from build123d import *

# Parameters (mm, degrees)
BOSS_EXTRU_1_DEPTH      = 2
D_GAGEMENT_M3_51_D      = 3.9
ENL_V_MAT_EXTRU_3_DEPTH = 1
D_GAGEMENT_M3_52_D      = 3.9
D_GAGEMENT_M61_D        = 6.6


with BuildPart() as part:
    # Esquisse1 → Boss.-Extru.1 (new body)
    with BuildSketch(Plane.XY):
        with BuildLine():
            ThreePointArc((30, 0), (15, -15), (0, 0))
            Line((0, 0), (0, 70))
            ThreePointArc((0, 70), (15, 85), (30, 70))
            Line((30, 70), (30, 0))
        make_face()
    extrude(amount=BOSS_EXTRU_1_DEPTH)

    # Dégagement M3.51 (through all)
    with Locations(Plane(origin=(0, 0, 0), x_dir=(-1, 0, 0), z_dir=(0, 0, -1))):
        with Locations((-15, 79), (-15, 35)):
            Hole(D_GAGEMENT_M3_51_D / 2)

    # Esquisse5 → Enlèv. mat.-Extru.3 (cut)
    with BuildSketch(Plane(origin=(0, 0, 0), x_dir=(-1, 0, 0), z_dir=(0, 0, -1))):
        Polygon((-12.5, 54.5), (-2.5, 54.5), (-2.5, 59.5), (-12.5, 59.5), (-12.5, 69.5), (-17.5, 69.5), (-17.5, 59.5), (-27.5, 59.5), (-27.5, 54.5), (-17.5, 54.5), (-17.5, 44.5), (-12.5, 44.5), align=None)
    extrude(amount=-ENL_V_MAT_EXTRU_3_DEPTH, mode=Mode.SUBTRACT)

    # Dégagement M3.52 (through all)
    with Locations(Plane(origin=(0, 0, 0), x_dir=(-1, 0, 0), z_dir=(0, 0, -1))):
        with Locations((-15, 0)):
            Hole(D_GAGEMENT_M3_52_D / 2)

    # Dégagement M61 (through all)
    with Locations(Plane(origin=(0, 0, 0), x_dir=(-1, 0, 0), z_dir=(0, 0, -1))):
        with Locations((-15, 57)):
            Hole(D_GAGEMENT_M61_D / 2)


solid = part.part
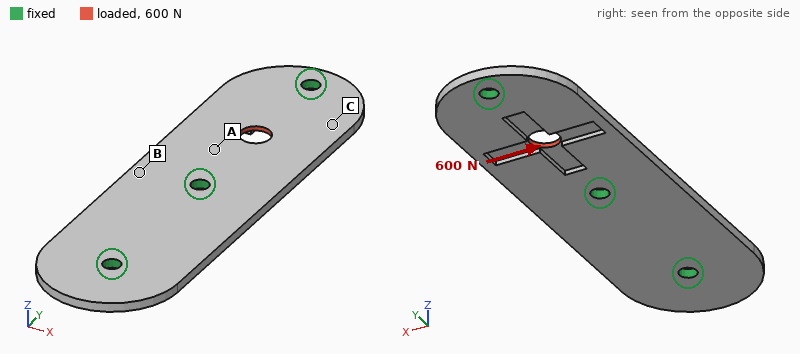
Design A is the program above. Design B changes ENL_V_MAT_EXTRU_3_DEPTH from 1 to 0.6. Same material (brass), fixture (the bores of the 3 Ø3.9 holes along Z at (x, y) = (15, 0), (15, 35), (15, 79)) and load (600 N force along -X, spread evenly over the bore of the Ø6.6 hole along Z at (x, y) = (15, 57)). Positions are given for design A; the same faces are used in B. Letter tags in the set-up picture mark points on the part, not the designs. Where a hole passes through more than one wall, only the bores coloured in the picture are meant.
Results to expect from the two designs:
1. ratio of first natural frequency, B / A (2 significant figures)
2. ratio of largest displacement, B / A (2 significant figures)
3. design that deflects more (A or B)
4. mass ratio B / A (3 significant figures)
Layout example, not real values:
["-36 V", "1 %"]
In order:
["1.0", "0.65", "A", "1.01"]
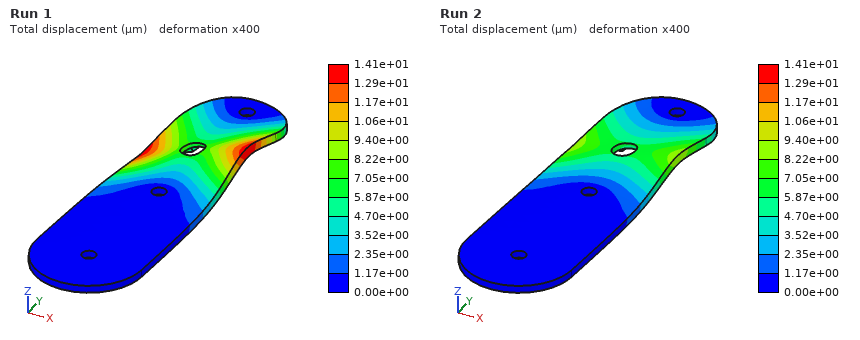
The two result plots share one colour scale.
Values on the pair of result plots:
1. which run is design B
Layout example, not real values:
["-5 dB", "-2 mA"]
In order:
["Run 2"]
